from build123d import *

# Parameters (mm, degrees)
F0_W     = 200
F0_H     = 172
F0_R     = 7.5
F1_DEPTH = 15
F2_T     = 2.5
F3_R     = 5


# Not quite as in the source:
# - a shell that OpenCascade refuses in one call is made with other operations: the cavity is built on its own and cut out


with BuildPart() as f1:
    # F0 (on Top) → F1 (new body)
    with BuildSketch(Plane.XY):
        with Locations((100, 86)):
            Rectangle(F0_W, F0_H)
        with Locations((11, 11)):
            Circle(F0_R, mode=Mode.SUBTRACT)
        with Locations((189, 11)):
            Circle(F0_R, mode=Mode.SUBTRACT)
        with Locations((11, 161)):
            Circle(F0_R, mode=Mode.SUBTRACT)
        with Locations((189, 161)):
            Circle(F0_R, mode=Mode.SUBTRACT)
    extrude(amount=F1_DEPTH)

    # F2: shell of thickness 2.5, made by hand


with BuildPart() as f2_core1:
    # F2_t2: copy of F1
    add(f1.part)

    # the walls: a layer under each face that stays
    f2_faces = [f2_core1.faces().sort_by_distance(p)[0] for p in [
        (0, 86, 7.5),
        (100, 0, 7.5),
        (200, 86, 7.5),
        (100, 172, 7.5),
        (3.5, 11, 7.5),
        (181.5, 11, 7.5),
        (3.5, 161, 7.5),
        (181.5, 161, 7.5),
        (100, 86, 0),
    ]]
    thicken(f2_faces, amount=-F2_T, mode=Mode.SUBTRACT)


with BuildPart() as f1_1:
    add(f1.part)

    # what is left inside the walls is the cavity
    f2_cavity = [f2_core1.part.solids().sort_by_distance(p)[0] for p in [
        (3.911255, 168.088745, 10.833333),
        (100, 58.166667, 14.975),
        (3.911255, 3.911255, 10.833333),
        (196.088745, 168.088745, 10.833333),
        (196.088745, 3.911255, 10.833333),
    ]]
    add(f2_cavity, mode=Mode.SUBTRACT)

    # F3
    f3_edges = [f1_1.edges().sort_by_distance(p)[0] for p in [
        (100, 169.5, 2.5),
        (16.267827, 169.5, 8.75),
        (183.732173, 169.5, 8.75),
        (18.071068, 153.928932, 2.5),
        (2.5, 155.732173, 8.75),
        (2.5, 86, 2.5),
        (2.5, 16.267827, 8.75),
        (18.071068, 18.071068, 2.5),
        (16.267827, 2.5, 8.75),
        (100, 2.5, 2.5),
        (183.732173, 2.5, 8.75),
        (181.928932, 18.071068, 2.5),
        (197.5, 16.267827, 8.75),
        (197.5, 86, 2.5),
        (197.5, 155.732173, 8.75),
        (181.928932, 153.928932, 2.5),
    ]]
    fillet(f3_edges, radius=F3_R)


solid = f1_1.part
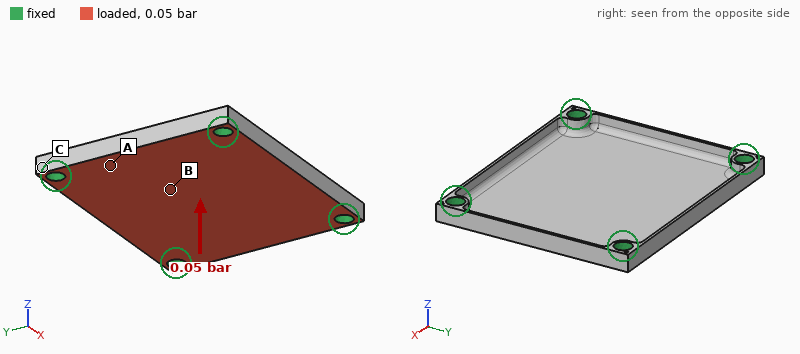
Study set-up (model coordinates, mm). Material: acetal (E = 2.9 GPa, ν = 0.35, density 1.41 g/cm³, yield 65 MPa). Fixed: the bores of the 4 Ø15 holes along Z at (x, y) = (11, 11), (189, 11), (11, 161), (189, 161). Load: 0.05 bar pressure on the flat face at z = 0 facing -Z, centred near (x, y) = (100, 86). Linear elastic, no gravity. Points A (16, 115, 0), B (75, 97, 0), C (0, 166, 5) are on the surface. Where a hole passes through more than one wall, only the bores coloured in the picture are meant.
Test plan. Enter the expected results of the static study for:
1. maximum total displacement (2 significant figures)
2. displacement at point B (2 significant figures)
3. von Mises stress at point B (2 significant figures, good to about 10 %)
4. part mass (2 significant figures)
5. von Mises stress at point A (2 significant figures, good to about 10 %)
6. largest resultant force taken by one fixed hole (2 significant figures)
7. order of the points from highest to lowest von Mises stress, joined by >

2.8 mm
2.4 mm
4.7 MPa
170 g
2.8 MPa
54 N
B > A > C
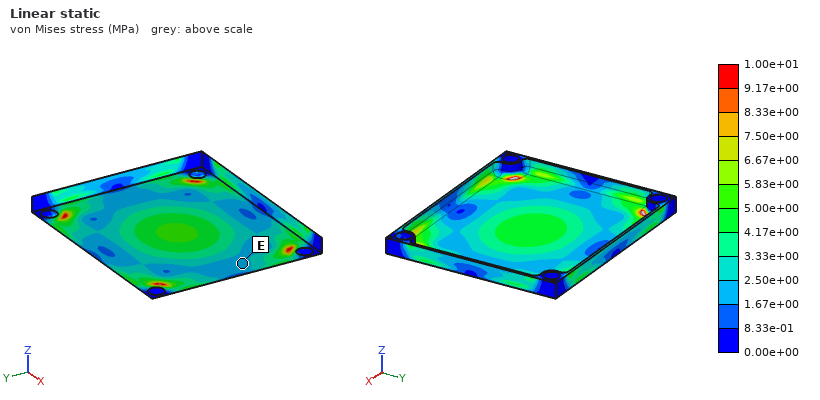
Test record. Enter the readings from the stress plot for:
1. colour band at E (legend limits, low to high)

1.67e+00 to 2.50e+00 MPa
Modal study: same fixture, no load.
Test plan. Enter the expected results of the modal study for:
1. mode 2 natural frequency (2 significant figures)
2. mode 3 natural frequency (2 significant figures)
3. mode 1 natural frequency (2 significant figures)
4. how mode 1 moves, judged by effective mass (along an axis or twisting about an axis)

300 Hz
330 Hz
140 Hz
along Z
